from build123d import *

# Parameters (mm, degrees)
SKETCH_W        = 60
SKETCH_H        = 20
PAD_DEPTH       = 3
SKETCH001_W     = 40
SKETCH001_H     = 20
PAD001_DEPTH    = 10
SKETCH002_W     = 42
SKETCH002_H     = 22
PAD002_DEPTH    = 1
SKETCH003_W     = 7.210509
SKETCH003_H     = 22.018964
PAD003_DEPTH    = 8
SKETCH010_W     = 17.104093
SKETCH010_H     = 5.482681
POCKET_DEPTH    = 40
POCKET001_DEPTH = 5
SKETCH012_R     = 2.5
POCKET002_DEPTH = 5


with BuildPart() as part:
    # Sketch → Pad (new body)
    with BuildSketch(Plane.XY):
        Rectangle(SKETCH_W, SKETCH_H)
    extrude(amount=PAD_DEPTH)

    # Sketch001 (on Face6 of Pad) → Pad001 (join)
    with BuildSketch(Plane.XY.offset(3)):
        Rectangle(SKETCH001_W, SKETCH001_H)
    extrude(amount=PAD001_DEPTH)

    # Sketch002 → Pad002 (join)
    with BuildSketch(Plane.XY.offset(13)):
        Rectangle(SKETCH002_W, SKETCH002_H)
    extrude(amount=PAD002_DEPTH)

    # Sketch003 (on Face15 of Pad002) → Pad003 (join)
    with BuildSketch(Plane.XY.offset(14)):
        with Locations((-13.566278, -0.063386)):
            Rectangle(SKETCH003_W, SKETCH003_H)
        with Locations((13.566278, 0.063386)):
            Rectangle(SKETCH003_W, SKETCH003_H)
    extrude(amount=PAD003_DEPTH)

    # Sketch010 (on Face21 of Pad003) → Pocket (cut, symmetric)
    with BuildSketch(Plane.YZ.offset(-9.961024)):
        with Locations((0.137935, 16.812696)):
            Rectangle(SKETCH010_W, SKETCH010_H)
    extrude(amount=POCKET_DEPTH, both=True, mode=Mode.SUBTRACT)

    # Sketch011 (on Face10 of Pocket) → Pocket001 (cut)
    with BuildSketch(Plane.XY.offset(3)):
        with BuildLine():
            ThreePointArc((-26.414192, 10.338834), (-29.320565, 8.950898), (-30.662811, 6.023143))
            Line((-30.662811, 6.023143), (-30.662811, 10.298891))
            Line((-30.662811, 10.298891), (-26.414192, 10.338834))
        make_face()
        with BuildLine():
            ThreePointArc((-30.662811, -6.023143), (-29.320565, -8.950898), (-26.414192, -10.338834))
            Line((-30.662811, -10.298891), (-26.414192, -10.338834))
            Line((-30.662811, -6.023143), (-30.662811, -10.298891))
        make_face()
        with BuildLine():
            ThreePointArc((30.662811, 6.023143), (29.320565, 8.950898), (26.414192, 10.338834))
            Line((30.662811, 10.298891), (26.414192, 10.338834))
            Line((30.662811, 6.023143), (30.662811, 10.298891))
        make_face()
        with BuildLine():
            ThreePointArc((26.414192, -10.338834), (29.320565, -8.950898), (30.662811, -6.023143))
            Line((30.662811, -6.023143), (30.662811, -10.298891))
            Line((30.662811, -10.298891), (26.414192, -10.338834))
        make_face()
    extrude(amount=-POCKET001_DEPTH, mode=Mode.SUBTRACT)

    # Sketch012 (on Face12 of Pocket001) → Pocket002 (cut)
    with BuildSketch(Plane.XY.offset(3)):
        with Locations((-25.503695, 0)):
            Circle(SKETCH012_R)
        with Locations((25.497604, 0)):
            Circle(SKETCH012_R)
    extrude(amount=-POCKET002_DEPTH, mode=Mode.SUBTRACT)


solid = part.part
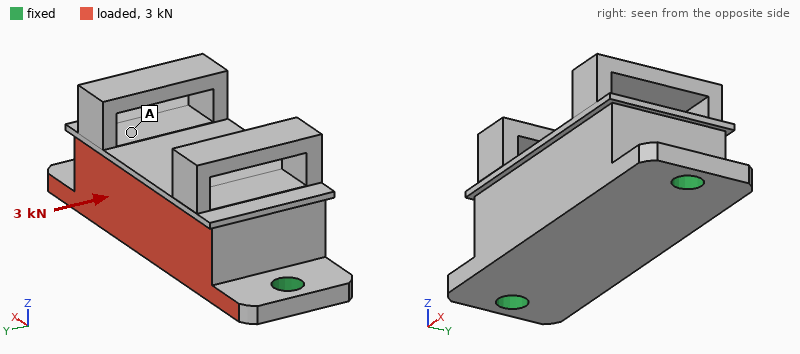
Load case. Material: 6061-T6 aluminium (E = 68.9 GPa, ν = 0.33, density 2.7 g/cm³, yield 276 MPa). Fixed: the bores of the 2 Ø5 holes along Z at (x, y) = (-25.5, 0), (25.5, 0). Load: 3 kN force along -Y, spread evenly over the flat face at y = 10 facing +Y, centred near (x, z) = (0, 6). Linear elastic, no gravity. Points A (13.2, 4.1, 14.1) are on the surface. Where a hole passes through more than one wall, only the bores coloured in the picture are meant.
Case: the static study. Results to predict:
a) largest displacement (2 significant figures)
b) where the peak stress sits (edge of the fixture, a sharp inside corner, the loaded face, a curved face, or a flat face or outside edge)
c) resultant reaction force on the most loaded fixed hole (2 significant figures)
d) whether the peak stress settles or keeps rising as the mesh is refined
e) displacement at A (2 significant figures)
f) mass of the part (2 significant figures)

0.14 mm
edge of the fixture
1.5 kN
keeps rising
0.088 mm
37 g
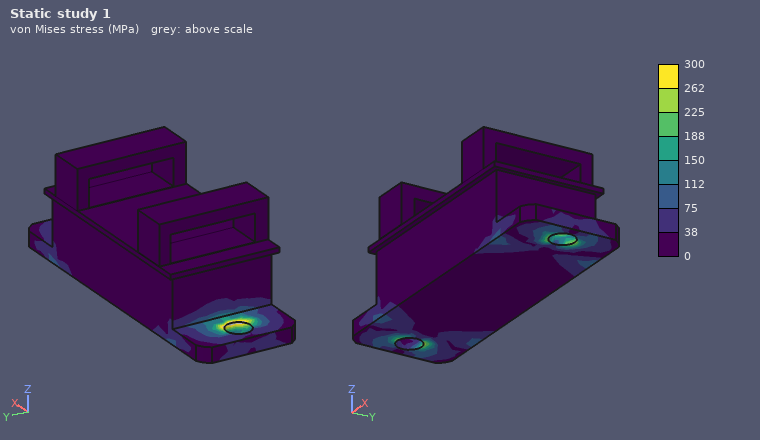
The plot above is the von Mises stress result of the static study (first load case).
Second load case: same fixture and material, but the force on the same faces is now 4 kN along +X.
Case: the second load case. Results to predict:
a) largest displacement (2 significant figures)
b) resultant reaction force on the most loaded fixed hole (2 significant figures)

15 µm
2.2 kN
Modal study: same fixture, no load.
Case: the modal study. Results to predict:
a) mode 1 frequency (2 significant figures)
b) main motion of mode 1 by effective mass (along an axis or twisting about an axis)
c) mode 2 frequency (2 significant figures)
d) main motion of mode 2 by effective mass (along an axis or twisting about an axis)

3900 Hz
along Y
9500 Hz
along Z
